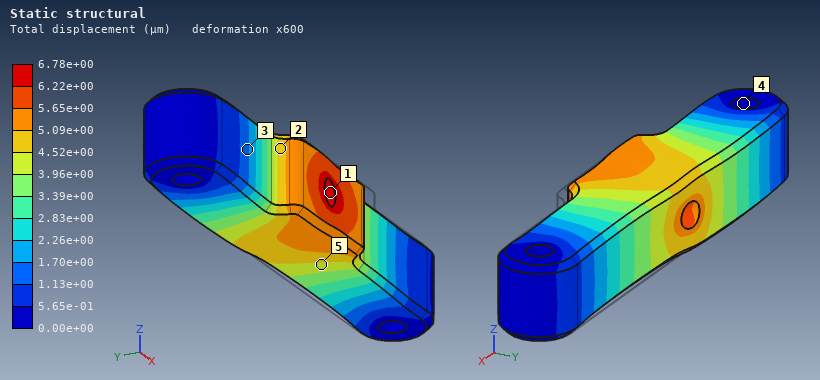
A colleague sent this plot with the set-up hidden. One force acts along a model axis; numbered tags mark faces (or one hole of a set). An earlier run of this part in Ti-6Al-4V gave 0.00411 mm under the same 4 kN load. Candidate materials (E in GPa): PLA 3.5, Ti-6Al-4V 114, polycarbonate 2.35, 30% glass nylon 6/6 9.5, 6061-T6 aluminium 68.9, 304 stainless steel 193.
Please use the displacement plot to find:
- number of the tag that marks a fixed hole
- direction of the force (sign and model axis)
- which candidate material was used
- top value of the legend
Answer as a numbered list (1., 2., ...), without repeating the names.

1. 4
2. -X
3. 6061-T6 aluminium
4. 6.78e+00 µm
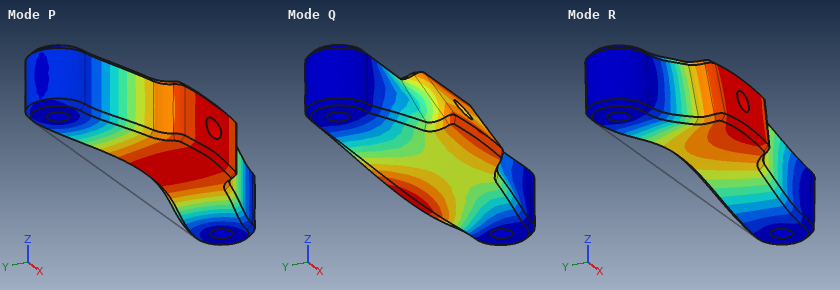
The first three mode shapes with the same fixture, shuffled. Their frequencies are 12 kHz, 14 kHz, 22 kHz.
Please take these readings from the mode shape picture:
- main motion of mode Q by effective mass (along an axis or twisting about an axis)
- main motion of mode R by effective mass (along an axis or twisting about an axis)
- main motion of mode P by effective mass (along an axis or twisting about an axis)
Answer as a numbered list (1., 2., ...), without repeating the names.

1. twisting about X
2. along Z
3. along Y
